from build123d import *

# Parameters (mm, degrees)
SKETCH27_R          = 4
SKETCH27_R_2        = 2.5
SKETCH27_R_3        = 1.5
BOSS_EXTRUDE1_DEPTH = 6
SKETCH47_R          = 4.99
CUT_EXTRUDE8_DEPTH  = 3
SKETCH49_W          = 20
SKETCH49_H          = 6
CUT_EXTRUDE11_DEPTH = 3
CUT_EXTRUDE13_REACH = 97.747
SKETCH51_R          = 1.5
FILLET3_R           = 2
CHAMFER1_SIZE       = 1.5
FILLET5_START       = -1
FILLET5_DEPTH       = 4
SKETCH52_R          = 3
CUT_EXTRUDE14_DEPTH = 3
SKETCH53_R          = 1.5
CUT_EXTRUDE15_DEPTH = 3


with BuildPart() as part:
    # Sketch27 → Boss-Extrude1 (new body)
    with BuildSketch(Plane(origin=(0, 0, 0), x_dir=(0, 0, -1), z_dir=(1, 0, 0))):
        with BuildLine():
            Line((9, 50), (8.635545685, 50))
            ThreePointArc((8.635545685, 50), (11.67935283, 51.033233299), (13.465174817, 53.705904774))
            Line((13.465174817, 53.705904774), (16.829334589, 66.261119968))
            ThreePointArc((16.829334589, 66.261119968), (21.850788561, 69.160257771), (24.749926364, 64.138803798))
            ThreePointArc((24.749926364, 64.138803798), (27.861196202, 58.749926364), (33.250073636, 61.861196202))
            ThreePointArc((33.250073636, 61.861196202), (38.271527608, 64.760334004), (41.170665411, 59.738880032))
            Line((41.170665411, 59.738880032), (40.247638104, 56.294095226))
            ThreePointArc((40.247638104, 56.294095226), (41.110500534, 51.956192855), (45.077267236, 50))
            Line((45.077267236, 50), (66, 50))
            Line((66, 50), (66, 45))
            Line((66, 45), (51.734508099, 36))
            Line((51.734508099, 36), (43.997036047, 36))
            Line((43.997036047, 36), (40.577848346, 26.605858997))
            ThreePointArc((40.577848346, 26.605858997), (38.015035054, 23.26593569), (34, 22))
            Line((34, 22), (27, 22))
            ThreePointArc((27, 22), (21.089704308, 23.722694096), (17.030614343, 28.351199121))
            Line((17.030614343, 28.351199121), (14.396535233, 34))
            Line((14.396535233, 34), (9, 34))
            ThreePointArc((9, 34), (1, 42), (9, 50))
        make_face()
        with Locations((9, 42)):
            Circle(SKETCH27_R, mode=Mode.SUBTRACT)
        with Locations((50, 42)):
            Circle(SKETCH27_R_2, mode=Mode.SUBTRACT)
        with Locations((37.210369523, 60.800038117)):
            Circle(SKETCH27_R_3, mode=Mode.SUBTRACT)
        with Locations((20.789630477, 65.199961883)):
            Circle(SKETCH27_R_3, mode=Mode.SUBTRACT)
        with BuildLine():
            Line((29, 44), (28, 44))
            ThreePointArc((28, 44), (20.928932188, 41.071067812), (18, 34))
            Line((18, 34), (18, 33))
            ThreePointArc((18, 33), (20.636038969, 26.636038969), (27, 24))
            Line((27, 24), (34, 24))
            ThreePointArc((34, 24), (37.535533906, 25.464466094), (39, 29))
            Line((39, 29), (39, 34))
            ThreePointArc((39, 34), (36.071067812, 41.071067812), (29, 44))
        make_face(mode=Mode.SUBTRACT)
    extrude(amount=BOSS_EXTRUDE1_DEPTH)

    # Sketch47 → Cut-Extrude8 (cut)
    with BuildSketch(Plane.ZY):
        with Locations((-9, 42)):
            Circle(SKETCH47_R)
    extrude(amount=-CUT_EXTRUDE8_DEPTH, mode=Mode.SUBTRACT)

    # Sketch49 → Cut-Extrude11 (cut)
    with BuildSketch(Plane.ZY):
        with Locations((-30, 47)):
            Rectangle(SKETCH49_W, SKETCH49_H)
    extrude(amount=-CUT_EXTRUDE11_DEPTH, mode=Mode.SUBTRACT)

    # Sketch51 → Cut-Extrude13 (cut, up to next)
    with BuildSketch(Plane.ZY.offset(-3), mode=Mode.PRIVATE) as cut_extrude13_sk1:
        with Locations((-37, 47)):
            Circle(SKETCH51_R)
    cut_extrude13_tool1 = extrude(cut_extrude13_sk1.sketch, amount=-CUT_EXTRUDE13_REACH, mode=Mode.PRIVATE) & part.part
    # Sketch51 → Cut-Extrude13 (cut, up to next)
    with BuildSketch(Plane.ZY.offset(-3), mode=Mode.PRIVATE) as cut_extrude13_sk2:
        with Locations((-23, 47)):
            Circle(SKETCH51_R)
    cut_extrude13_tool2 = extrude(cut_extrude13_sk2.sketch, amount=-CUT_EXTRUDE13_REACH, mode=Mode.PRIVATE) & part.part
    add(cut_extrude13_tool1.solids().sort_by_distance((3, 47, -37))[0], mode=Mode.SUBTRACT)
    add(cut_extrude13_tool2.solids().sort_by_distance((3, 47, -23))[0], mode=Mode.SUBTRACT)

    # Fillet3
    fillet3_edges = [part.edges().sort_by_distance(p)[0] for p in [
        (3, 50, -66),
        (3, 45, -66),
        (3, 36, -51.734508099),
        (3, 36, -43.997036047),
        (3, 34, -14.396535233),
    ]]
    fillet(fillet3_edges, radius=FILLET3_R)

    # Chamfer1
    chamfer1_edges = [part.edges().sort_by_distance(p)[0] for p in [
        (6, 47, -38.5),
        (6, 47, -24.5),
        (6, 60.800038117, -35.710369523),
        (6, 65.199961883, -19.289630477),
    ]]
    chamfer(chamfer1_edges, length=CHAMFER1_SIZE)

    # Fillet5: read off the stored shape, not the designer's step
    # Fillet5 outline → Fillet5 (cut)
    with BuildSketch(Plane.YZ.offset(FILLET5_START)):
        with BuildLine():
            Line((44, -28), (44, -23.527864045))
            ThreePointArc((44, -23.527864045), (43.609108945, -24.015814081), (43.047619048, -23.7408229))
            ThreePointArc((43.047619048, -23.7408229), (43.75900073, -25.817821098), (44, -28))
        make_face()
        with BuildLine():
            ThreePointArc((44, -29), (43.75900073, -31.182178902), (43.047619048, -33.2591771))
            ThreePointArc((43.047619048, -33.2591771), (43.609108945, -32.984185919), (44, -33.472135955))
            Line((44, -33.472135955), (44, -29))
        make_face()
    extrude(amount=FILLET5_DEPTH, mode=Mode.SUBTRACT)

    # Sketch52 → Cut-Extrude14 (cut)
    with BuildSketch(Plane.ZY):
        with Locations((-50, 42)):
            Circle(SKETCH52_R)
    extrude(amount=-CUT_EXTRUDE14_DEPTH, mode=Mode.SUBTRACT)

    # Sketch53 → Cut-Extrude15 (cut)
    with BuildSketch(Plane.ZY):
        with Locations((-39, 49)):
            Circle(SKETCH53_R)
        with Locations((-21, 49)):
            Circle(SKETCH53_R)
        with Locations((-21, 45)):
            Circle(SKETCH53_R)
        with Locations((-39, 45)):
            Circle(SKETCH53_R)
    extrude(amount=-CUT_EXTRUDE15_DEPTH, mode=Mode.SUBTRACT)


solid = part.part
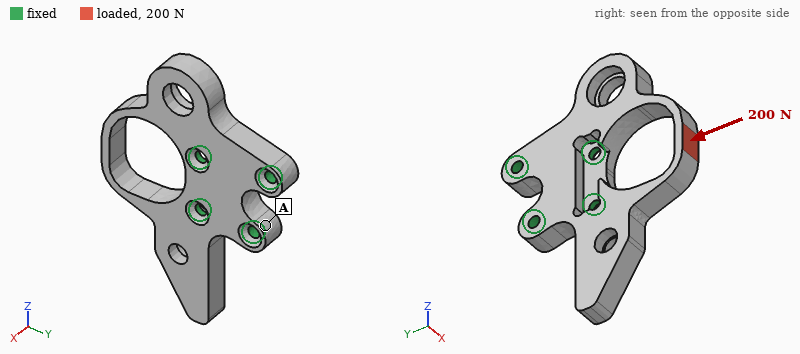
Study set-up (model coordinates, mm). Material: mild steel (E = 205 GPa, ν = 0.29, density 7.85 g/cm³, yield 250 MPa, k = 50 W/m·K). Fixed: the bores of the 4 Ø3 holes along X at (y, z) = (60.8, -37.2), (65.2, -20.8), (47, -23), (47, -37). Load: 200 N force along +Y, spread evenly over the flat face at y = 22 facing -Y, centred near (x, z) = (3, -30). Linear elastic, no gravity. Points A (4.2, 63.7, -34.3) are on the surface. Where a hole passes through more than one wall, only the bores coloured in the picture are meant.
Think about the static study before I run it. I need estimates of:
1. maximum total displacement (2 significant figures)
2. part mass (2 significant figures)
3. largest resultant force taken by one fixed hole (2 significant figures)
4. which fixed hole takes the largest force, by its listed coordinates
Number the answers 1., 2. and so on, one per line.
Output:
1. 11 µm
2. 48 g
3. 150 N
4. (47, -37)
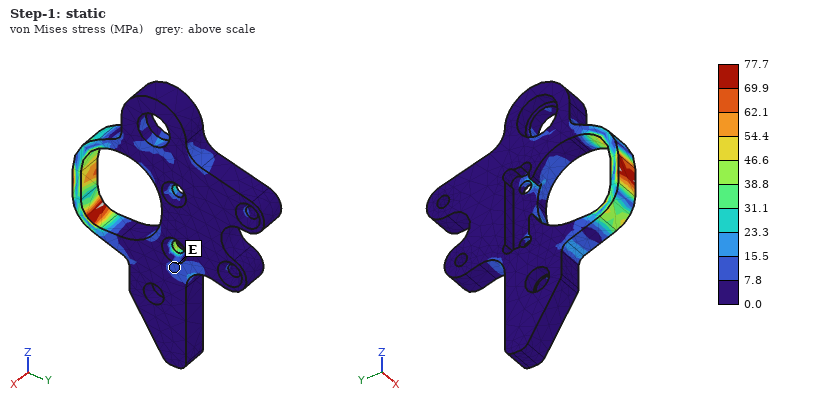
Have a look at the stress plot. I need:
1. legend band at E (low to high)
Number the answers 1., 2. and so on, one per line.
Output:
1. 7.8 to 15.5 MPa
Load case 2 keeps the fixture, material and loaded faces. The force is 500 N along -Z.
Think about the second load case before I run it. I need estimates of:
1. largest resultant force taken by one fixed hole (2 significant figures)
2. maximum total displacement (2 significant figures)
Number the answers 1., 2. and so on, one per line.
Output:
1. 470 N
2. 32 µm
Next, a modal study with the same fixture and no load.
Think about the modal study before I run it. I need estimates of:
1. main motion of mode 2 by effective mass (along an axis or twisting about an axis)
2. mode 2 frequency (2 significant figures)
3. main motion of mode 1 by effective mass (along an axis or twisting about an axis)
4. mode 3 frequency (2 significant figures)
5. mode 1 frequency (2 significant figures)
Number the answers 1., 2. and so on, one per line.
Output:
1. along X
2. 5900 Hz
3. along X
4. 7300 Hz
5. 4200 Hz
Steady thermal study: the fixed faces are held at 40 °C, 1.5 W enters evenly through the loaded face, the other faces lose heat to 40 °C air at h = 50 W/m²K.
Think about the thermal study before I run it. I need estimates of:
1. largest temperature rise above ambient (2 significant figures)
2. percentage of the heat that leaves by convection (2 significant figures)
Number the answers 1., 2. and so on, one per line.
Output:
1. 21 K
2. 36 %
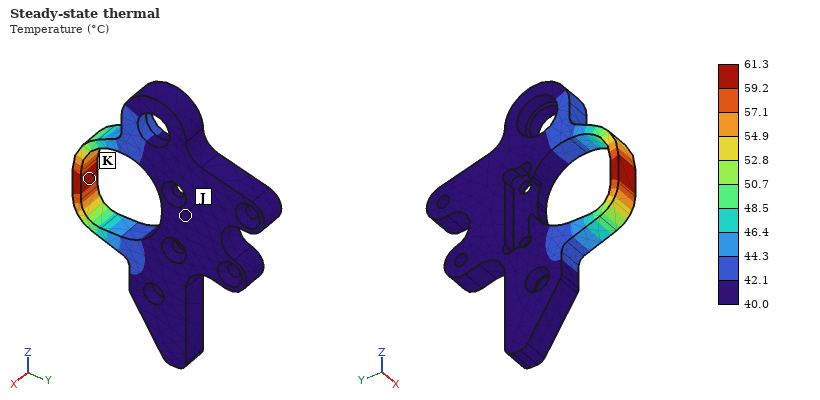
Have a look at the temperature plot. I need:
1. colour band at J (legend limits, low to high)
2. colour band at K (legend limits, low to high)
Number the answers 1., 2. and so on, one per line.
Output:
1. 40.0 to 42.1 °C
2. 59.2 to 61.3 °C
